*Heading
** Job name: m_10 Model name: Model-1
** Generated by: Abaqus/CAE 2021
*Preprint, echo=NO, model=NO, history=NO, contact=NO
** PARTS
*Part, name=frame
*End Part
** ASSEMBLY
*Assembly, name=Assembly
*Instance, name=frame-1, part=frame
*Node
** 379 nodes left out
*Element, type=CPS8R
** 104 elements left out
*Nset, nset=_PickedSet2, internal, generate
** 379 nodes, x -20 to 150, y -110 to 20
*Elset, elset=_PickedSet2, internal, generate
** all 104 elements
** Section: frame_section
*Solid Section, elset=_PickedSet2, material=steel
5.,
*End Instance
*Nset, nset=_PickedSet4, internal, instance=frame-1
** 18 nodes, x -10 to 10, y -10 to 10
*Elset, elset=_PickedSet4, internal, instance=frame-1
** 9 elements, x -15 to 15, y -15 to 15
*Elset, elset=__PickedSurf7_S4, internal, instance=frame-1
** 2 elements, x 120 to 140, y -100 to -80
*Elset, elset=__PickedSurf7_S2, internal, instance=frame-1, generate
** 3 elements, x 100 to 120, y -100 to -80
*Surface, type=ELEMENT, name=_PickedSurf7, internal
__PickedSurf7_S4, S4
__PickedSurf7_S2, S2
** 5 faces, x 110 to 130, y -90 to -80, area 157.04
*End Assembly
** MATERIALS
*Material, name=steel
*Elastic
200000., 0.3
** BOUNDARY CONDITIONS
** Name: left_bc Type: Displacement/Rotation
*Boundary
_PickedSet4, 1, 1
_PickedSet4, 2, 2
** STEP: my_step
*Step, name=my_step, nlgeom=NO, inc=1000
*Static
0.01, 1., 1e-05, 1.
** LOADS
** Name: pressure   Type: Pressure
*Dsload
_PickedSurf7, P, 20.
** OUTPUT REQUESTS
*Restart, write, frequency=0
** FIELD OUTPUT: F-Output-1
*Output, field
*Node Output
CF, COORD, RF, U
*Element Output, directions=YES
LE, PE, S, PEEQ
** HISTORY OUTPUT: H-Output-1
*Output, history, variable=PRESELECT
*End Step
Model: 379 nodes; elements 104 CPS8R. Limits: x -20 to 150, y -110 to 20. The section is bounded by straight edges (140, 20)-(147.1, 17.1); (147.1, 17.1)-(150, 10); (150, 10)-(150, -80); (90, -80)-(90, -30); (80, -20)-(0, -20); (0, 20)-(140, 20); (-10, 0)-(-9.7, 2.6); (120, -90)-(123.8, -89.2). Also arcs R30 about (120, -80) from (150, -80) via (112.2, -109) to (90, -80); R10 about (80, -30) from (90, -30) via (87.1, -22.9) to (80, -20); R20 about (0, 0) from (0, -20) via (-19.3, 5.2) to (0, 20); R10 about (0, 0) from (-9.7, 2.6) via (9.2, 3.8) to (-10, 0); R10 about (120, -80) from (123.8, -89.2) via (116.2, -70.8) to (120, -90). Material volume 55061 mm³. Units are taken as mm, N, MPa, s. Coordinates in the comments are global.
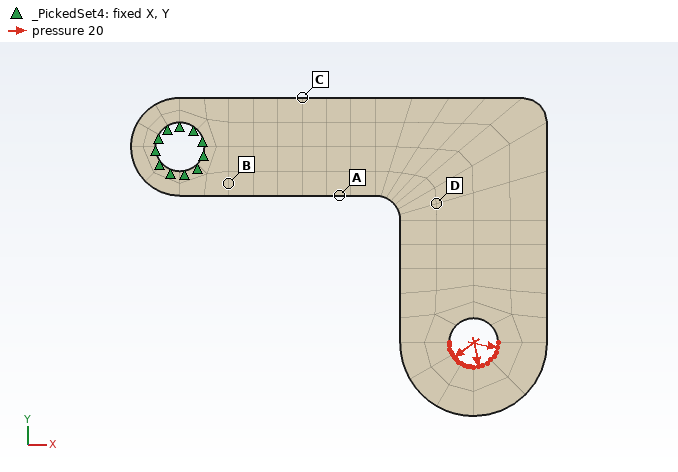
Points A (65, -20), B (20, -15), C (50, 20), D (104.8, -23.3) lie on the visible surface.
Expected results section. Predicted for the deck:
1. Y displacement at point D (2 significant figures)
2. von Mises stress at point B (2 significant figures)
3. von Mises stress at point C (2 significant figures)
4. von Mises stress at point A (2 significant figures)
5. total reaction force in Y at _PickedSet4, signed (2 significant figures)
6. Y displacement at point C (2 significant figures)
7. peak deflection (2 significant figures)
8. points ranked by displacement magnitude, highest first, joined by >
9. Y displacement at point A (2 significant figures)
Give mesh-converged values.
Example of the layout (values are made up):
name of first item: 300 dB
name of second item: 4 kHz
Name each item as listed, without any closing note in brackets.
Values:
Y displacement at point D: -0.20 mm
von Mises stress at point B: 110 MPa
von Mises stress at point C: 100 MPa
von Mises stress at point A: 83 MPa
total reaction force in Y at _PickedSet4, signed: 2000 N
Y displacement at point C: -0.062 mm
peak deflection: 0.42 mm
points ranked by displacement magnitude, highest first, joined by >: D > A > C > B
Y displacement at point A: -0.095 mm
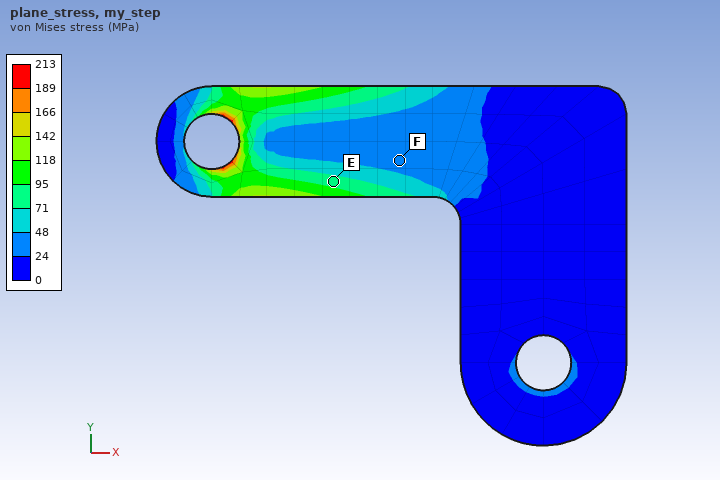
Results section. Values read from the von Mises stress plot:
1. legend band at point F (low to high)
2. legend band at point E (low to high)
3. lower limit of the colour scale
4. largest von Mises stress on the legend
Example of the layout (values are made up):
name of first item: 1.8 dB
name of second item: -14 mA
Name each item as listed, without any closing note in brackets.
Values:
legend band at point F: 24 to 48 MPa
legend band at point E: 71 to 95 MPa
lower limit of the colour scale: 0 MPa
largest von Mises stress on the legend: 213 MPa
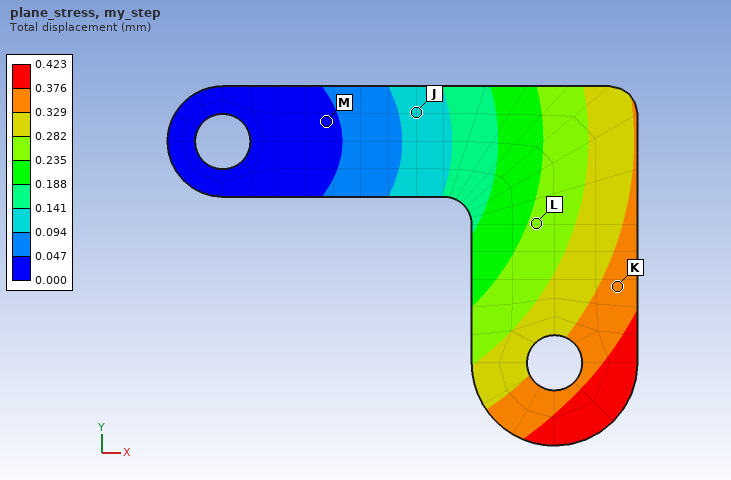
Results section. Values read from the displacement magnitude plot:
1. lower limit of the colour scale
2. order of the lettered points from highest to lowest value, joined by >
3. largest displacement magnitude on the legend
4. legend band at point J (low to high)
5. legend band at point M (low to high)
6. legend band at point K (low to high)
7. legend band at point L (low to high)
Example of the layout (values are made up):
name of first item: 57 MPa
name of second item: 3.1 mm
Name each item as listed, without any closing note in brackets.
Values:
lower limit of the colour scale: 0.000 mm
order of the lettered points from highest to lowest value, joined by >: K > L > J > M
largest displacement magnitude on the legend: 0.423 mm
legend band at point J: 0.094 to 0.141 mm
legend band at point M: 0.000 to 0.047 mm
legend band at point K: 0.329 to 0.376 mm
legend band at point L: 0.235 to 0.282 mm
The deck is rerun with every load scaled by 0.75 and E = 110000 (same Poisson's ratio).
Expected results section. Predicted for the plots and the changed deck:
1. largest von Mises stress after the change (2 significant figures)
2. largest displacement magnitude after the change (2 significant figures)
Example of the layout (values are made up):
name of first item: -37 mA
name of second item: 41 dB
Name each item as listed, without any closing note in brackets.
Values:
largest von Mises stress after the change: 160 MPa
largest displacement magnitude after the change: 0.58 mm
